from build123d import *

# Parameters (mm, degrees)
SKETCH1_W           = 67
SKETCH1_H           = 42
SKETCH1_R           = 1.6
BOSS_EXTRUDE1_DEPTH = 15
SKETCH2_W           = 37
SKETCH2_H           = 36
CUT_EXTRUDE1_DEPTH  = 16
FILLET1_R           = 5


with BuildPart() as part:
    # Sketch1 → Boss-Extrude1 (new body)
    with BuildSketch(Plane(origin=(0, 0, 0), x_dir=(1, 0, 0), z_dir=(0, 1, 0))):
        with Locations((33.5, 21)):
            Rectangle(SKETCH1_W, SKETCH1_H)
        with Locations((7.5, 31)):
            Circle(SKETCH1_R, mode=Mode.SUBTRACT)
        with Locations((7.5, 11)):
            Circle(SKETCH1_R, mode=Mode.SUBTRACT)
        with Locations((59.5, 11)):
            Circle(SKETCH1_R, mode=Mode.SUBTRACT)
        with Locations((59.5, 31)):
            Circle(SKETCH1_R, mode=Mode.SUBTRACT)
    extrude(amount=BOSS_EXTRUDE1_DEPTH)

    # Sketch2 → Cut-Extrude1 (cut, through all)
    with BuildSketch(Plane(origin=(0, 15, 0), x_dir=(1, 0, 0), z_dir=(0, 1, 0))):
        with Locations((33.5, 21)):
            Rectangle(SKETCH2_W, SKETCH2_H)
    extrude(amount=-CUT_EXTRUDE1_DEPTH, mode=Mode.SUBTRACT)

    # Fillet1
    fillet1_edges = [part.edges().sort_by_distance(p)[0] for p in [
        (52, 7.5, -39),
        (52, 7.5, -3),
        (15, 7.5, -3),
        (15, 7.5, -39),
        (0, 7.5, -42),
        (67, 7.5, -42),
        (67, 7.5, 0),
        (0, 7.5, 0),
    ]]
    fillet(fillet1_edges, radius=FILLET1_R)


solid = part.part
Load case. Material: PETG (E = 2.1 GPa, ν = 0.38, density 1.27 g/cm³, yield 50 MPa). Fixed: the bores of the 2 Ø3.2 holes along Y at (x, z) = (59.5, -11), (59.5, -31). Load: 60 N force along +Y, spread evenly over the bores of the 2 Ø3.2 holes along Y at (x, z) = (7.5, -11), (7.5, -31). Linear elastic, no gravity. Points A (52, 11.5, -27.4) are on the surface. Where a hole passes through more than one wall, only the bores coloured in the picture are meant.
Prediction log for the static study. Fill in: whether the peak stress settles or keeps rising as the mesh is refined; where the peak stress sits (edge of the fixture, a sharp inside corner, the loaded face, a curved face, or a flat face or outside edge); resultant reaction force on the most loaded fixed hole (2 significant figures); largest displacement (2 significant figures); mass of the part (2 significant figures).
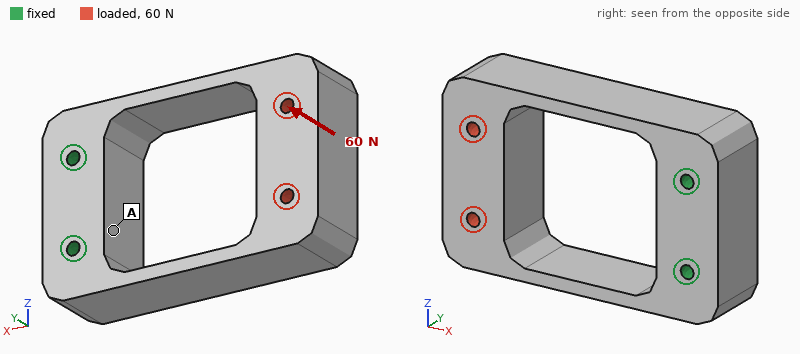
keeps rising
a sharp inside corner
30 N
0.94 mm
28 g
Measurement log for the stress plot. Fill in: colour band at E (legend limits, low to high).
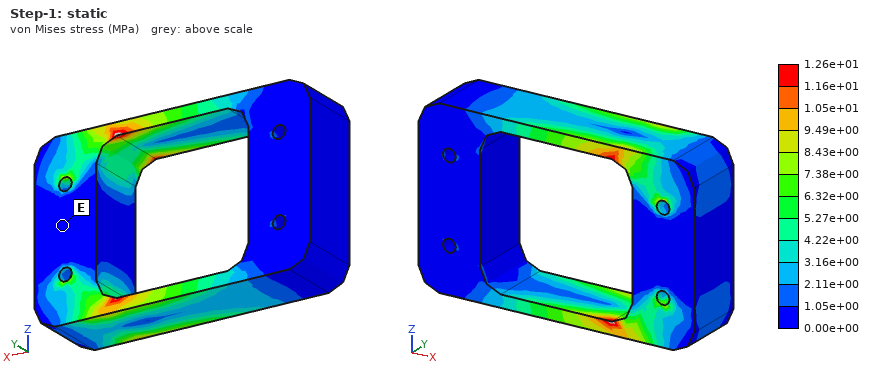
0.00e+00 to 1.05e+00 MPa
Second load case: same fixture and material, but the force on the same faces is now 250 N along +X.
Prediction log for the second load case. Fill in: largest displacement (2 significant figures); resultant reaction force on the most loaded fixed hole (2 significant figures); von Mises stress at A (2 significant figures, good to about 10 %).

0.11 mm
130 N
1.6 MPa
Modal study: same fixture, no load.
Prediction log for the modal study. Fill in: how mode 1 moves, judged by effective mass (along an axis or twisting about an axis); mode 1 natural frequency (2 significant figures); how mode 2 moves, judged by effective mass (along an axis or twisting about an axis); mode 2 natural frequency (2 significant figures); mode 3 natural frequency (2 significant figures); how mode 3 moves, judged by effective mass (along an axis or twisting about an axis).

along Z
280 Hz
along Y
400 Hz
1000 Hz
twisting about X
